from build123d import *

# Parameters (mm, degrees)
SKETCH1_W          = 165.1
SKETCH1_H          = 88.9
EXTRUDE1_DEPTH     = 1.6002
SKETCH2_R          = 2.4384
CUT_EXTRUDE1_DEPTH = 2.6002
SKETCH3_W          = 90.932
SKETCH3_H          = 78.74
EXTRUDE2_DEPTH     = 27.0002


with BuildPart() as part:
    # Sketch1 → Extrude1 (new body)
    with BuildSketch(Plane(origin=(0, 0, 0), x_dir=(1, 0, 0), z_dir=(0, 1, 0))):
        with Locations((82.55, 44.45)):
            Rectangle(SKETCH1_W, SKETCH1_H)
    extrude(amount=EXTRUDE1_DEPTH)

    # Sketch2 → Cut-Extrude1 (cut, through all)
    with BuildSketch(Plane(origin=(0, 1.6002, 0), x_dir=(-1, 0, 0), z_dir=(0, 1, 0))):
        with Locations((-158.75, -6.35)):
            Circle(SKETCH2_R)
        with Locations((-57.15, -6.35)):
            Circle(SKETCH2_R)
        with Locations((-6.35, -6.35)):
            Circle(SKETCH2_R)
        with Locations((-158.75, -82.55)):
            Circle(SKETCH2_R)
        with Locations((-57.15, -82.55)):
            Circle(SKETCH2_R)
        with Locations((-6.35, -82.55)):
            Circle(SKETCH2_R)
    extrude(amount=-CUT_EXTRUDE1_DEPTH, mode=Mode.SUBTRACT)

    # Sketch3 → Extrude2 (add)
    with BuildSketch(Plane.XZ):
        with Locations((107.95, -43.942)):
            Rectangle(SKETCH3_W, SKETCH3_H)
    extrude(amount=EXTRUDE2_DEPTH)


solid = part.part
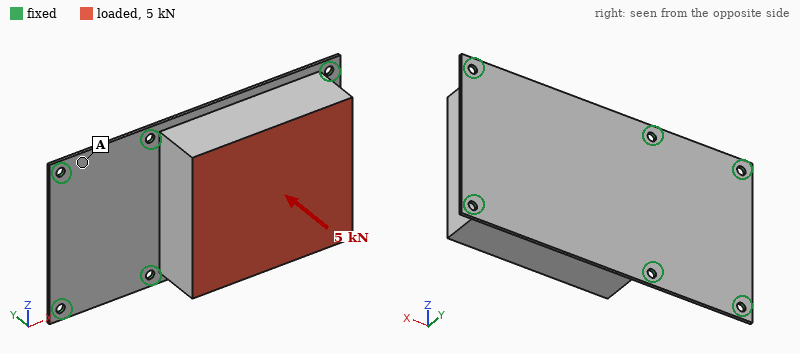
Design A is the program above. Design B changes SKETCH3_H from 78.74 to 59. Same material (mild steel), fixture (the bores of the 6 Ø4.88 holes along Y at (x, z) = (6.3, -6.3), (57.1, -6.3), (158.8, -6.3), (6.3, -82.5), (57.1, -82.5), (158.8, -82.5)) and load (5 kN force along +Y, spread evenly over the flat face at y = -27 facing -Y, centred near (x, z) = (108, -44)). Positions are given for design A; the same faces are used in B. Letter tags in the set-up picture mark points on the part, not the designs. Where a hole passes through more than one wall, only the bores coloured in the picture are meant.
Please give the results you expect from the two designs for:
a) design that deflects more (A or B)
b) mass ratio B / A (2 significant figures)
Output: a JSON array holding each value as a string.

["B", "0.78"]
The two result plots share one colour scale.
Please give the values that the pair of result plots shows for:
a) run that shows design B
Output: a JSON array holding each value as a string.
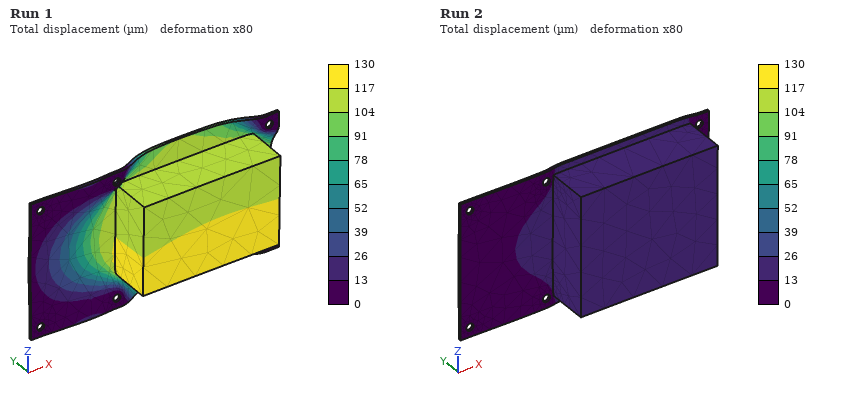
["Run 1"]
